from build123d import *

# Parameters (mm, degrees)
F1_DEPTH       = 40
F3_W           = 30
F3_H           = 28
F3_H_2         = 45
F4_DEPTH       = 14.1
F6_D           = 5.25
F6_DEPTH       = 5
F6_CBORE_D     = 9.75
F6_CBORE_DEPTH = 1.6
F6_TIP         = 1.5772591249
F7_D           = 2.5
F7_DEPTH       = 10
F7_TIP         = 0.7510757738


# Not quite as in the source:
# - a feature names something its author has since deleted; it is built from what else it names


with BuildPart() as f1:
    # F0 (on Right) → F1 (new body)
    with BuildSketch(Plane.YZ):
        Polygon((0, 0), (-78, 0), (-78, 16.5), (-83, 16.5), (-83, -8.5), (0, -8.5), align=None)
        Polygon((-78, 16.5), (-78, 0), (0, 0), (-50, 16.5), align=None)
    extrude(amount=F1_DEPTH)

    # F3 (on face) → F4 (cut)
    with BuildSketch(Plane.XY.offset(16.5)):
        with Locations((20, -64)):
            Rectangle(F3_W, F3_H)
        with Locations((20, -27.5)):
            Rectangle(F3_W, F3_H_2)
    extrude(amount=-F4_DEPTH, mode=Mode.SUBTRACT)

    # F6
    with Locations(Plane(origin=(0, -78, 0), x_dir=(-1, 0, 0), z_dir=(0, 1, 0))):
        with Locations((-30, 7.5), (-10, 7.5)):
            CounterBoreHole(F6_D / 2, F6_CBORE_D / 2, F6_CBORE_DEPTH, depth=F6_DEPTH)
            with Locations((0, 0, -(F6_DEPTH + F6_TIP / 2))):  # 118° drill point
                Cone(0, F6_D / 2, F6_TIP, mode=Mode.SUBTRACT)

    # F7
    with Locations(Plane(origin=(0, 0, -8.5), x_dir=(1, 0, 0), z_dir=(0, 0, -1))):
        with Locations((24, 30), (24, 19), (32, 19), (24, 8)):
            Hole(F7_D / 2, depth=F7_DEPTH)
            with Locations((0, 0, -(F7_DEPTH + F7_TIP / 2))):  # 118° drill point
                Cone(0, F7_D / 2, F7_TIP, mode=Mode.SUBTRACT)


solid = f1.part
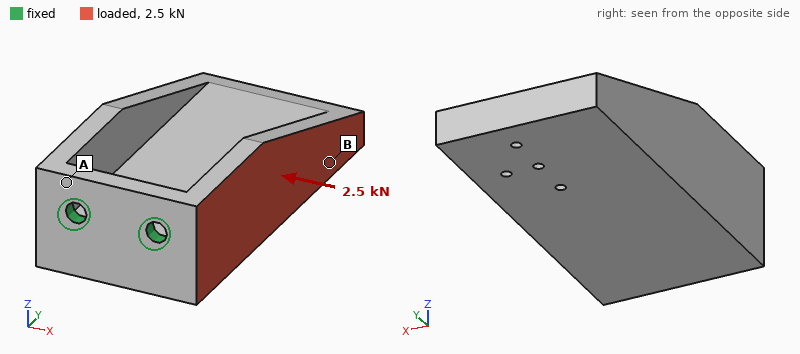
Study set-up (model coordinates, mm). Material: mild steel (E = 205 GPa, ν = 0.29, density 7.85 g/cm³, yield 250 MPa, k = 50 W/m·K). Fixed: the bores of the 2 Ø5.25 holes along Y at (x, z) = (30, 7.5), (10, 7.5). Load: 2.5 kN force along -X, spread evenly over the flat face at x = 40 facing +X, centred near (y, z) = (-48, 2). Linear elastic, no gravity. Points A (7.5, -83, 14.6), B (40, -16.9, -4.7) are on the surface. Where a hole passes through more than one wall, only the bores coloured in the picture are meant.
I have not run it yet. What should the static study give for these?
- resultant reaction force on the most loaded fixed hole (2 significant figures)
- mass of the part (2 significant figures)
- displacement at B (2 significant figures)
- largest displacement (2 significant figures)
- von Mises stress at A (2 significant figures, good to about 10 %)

3.7 kN
350 g
54 µm
70 µm
57 MPa
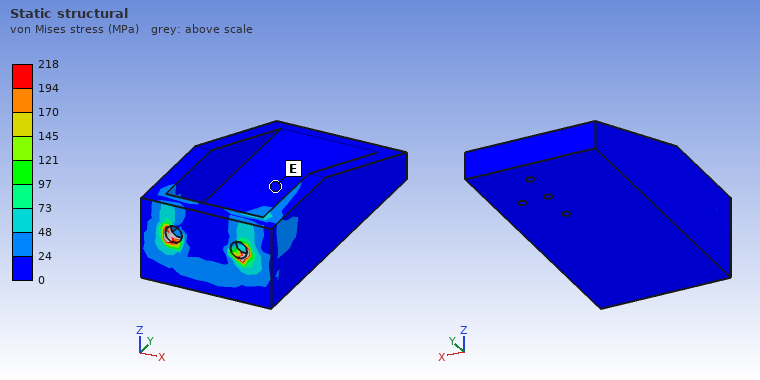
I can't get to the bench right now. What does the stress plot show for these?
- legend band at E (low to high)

0 to 24 MPa
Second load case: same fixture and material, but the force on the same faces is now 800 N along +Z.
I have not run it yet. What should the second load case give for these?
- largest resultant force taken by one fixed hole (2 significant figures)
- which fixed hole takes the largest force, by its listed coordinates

1.1 kN
(30, 7.5)
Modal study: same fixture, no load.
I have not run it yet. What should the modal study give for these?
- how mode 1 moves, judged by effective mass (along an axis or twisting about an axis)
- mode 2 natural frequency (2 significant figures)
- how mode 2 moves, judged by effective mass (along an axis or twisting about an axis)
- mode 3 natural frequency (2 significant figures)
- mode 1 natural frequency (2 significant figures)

along Z
2000 Hz
along X
4700 Hz
800 Hz
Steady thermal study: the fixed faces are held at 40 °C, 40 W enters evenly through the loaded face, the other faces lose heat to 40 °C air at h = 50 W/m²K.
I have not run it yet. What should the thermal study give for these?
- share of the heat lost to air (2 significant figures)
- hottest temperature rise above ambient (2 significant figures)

41 %
49 K
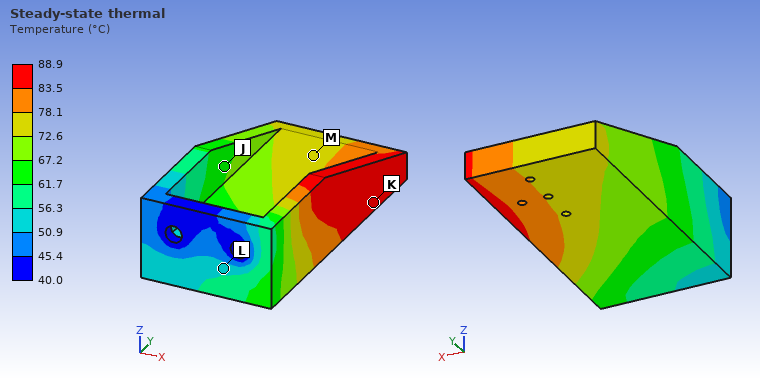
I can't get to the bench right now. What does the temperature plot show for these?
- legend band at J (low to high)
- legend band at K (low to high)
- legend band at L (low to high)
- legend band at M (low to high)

61.7 to 67.2 °C
83.5 to 88.9 °C
50.9 to 56.3 °C
72.6 to 78.1 °C
